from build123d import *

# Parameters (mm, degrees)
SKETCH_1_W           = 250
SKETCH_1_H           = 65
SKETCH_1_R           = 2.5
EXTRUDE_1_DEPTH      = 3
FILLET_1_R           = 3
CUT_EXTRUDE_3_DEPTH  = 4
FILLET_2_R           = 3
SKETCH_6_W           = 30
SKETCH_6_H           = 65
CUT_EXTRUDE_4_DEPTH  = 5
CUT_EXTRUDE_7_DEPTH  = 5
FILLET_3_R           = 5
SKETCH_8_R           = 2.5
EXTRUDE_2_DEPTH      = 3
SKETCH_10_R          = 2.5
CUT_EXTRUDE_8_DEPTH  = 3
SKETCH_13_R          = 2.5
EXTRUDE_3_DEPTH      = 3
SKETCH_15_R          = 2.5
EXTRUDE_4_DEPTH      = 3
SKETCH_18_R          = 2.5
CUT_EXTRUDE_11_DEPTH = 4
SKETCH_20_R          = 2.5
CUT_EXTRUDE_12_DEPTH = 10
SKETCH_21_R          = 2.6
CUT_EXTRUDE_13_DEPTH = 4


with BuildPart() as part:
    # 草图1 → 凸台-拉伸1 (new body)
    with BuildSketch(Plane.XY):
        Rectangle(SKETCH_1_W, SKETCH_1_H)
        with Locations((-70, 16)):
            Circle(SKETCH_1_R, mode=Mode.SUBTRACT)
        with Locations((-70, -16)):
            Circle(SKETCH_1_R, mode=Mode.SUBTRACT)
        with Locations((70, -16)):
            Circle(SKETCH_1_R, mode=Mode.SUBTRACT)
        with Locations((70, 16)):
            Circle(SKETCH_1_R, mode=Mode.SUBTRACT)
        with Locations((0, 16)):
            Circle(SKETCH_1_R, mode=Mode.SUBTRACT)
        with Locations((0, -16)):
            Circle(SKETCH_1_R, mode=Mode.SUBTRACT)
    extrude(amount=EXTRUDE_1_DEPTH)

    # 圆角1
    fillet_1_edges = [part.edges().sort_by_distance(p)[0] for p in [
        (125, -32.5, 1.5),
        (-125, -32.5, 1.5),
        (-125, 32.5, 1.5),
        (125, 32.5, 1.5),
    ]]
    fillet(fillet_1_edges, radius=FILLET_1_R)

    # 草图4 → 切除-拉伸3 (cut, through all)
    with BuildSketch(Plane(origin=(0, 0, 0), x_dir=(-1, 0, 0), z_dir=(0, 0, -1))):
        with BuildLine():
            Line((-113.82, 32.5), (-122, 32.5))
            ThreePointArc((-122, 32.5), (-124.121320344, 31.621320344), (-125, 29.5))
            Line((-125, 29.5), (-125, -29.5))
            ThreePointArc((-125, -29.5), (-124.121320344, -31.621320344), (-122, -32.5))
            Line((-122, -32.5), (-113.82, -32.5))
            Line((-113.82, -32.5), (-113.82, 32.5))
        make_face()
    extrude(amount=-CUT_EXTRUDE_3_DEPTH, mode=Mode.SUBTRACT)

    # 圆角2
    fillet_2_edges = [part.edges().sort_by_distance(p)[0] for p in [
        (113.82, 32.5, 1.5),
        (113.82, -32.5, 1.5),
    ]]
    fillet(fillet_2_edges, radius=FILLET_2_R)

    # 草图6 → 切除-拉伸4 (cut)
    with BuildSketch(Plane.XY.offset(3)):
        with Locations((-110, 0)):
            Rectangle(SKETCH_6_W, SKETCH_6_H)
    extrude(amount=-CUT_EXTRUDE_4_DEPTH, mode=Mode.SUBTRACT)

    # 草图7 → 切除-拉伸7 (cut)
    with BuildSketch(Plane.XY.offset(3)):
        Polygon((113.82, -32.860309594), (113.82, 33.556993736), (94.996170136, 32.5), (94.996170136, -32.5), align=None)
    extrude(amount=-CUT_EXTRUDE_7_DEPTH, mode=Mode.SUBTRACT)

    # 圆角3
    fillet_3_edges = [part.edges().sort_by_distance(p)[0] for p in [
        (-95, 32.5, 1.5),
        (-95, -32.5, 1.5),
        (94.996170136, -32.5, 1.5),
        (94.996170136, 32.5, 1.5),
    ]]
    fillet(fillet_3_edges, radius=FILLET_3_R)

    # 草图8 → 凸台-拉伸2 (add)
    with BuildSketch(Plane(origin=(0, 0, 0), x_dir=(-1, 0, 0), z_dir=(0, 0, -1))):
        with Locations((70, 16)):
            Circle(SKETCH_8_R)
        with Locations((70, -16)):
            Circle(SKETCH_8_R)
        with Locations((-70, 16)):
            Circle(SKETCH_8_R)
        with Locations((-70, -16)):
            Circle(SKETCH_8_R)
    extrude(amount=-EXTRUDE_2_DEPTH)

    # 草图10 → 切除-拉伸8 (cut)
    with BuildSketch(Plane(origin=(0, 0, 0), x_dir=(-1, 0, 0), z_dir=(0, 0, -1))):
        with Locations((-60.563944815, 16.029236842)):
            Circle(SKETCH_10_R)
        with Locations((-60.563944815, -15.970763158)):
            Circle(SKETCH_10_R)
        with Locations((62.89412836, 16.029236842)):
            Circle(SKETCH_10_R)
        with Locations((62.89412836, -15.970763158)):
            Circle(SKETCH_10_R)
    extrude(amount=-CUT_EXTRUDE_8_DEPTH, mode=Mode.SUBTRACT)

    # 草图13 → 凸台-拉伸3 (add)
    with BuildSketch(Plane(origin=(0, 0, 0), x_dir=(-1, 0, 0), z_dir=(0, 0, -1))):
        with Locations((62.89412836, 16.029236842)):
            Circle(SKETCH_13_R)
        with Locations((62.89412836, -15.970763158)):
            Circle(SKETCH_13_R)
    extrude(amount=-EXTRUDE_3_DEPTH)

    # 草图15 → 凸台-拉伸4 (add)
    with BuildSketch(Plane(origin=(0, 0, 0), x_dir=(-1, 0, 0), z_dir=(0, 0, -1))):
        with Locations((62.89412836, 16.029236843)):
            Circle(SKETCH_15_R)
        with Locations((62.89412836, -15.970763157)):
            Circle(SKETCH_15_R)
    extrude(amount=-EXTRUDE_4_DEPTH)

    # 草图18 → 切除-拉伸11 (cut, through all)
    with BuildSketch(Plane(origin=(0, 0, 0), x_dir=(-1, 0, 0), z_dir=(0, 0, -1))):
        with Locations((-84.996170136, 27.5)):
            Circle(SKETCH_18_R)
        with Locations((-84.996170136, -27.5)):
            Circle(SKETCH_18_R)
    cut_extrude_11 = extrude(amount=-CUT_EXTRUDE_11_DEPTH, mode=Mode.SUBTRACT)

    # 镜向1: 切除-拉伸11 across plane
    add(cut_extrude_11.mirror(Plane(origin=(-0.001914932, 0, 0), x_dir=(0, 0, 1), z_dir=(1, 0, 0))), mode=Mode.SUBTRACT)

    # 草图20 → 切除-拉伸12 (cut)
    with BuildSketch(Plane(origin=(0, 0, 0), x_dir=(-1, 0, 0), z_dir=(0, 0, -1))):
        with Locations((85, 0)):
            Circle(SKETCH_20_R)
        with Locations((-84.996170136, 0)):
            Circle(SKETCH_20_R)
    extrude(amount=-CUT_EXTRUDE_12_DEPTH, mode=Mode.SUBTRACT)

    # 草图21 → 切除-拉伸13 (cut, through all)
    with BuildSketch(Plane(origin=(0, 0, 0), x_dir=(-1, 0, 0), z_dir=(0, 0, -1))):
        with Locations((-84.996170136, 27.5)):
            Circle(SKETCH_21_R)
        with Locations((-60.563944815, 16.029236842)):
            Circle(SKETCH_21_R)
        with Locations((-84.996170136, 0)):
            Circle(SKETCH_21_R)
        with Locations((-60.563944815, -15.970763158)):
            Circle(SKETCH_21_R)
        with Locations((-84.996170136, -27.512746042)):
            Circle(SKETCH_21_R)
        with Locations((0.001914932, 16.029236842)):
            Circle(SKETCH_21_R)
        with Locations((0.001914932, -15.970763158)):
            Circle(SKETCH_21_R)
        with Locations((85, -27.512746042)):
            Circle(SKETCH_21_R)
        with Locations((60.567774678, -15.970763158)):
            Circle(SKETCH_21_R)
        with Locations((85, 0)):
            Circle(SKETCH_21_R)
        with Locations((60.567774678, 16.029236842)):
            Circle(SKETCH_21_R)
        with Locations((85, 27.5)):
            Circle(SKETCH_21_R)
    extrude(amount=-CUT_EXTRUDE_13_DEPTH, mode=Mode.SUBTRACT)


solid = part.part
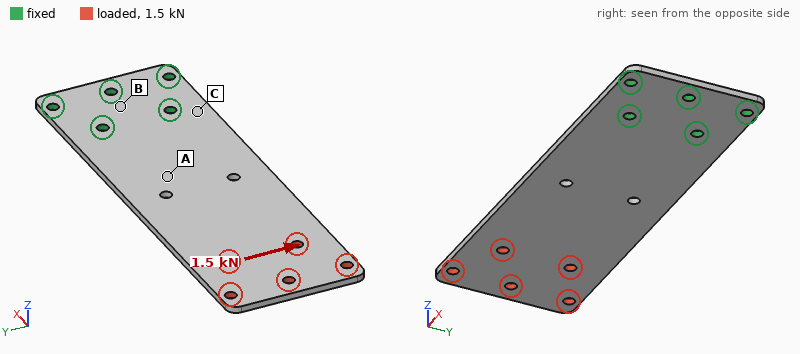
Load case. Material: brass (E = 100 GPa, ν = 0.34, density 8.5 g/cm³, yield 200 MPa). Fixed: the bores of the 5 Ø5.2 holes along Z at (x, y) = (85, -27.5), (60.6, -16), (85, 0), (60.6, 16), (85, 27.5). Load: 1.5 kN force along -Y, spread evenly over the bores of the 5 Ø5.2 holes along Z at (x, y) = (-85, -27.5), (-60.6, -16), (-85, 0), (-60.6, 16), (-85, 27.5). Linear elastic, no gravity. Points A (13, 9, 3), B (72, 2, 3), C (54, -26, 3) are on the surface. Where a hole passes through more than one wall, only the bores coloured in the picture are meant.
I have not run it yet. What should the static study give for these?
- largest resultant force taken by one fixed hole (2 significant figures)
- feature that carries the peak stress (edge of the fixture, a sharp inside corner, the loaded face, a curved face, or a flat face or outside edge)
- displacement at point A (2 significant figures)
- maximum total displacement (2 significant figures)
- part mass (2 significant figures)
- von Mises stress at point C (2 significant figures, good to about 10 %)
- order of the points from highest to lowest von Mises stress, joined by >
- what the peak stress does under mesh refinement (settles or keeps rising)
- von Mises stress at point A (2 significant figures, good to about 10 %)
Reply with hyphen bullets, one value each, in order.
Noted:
- 3.7 kN
- edge of the fixture
- 0.056 mm
- 0.31 mm
- 310 g
- 60 MPa
- C > A > B
- keeps rising
- 28 MPa
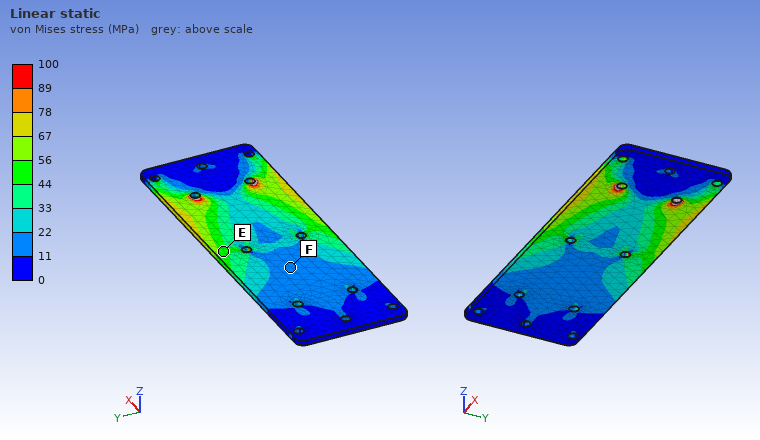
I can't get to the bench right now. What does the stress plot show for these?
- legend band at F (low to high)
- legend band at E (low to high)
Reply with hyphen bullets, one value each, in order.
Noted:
- 11 to 22 MPa
- 44 to 56 MPa
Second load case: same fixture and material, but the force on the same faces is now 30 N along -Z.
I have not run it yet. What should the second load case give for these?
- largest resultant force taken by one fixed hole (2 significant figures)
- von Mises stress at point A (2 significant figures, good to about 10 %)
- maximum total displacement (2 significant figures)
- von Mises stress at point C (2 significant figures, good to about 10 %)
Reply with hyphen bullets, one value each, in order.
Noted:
- 42 N
- 26 MPa
- 2.0 mm
- 33 MPa
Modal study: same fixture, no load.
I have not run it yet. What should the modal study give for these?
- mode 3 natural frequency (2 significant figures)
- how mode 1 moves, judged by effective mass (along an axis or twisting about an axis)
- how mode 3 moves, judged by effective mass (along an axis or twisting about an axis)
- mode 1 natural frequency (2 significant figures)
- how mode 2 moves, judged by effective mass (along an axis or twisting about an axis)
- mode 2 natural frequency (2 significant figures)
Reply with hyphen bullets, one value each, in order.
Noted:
- 440 Hz
- along Z
- along Z
- 71 Hz
- twisting about X
- 340 Hz
